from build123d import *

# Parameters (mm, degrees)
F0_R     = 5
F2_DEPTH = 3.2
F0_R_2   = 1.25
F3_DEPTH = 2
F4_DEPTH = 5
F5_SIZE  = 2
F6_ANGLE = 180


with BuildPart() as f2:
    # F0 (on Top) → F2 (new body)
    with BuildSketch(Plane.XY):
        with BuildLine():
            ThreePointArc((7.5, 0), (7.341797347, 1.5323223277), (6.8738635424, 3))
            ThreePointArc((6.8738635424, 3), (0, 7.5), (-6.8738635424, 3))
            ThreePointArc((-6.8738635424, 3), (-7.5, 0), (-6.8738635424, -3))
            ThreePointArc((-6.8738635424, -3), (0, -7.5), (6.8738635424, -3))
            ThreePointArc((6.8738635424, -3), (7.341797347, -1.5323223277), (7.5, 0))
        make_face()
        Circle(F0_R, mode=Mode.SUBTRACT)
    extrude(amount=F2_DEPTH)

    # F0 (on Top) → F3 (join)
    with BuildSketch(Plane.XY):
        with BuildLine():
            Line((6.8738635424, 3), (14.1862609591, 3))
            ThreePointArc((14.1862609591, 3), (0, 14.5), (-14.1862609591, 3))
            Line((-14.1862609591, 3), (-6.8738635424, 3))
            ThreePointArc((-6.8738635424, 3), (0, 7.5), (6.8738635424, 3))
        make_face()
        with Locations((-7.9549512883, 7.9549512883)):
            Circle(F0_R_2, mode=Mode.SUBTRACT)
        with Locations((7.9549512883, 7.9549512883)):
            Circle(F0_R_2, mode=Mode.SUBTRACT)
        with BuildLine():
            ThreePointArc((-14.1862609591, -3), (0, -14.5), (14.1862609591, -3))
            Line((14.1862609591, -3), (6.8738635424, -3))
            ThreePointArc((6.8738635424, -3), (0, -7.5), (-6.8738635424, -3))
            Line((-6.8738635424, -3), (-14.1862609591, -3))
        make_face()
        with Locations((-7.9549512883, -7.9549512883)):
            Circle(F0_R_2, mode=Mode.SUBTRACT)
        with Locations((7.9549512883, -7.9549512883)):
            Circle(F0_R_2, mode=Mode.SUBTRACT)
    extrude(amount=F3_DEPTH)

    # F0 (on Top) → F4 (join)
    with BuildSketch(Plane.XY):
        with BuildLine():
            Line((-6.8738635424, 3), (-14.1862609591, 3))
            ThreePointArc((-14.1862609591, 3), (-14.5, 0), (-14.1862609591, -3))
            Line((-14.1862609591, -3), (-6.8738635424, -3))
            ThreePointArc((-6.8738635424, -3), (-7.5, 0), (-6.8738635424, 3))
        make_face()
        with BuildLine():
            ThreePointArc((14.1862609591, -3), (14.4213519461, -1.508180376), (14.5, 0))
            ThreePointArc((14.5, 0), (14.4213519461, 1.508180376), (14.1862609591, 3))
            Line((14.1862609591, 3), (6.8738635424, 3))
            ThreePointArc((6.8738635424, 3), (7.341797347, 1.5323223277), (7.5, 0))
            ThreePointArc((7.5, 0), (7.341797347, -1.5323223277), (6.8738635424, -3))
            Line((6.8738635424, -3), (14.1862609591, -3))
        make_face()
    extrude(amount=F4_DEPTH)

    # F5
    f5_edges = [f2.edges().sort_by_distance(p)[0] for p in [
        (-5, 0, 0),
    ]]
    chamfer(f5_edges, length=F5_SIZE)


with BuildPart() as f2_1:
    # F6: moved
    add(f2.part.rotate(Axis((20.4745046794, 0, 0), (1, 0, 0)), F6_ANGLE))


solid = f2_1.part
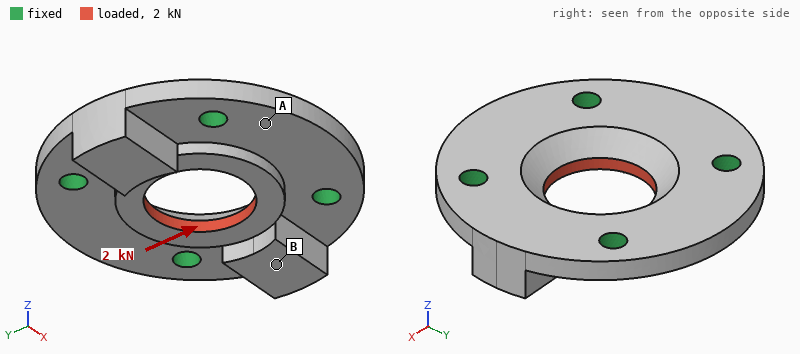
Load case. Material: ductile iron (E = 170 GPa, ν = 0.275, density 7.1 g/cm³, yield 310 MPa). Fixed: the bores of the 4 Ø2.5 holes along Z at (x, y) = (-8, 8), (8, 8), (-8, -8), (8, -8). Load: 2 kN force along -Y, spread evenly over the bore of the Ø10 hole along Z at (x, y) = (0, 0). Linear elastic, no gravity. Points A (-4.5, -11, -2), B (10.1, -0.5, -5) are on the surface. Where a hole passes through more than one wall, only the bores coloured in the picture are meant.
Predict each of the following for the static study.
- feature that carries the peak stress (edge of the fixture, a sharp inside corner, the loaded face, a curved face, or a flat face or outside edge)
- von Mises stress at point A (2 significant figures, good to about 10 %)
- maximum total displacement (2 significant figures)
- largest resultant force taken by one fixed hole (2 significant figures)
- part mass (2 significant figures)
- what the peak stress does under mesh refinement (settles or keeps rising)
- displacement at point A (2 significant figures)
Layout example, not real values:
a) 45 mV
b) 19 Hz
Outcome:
a) edge of the fixture
b) 24 MPa
c) 5.6 µm
d) 510 N
e) 10 g
f) keeps rising
g) 1.6 µm
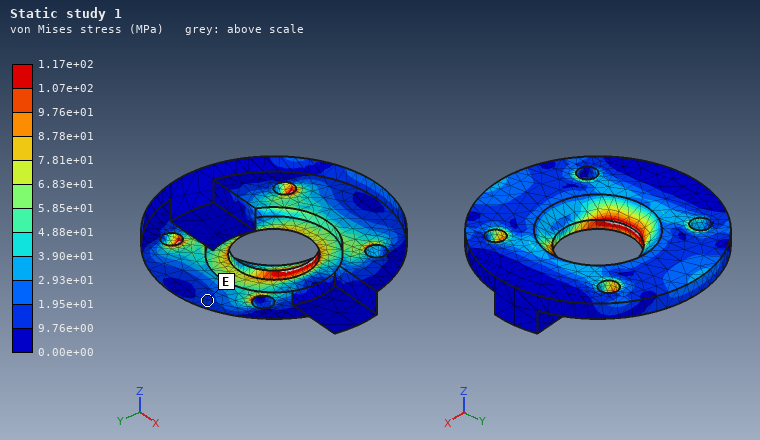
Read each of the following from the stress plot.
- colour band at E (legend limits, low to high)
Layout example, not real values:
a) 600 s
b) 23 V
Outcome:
a) 9.76e+00 to 1.95e+01 MPa
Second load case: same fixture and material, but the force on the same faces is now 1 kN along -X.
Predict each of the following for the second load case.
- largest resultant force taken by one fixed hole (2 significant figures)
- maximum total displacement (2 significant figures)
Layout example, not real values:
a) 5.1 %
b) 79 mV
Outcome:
a) 260 N
b) 2.7 µm
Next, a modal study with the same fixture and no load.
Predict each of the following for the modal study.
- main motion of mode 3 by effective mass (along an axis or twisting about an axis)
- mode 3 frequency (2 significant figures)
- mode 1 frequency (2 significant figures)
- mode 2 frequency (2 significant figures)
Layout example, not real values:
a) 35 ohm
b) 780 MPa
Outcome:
a) twisting about X
b) 31 kHz
c) 25 kHz
d) 25 kHz
